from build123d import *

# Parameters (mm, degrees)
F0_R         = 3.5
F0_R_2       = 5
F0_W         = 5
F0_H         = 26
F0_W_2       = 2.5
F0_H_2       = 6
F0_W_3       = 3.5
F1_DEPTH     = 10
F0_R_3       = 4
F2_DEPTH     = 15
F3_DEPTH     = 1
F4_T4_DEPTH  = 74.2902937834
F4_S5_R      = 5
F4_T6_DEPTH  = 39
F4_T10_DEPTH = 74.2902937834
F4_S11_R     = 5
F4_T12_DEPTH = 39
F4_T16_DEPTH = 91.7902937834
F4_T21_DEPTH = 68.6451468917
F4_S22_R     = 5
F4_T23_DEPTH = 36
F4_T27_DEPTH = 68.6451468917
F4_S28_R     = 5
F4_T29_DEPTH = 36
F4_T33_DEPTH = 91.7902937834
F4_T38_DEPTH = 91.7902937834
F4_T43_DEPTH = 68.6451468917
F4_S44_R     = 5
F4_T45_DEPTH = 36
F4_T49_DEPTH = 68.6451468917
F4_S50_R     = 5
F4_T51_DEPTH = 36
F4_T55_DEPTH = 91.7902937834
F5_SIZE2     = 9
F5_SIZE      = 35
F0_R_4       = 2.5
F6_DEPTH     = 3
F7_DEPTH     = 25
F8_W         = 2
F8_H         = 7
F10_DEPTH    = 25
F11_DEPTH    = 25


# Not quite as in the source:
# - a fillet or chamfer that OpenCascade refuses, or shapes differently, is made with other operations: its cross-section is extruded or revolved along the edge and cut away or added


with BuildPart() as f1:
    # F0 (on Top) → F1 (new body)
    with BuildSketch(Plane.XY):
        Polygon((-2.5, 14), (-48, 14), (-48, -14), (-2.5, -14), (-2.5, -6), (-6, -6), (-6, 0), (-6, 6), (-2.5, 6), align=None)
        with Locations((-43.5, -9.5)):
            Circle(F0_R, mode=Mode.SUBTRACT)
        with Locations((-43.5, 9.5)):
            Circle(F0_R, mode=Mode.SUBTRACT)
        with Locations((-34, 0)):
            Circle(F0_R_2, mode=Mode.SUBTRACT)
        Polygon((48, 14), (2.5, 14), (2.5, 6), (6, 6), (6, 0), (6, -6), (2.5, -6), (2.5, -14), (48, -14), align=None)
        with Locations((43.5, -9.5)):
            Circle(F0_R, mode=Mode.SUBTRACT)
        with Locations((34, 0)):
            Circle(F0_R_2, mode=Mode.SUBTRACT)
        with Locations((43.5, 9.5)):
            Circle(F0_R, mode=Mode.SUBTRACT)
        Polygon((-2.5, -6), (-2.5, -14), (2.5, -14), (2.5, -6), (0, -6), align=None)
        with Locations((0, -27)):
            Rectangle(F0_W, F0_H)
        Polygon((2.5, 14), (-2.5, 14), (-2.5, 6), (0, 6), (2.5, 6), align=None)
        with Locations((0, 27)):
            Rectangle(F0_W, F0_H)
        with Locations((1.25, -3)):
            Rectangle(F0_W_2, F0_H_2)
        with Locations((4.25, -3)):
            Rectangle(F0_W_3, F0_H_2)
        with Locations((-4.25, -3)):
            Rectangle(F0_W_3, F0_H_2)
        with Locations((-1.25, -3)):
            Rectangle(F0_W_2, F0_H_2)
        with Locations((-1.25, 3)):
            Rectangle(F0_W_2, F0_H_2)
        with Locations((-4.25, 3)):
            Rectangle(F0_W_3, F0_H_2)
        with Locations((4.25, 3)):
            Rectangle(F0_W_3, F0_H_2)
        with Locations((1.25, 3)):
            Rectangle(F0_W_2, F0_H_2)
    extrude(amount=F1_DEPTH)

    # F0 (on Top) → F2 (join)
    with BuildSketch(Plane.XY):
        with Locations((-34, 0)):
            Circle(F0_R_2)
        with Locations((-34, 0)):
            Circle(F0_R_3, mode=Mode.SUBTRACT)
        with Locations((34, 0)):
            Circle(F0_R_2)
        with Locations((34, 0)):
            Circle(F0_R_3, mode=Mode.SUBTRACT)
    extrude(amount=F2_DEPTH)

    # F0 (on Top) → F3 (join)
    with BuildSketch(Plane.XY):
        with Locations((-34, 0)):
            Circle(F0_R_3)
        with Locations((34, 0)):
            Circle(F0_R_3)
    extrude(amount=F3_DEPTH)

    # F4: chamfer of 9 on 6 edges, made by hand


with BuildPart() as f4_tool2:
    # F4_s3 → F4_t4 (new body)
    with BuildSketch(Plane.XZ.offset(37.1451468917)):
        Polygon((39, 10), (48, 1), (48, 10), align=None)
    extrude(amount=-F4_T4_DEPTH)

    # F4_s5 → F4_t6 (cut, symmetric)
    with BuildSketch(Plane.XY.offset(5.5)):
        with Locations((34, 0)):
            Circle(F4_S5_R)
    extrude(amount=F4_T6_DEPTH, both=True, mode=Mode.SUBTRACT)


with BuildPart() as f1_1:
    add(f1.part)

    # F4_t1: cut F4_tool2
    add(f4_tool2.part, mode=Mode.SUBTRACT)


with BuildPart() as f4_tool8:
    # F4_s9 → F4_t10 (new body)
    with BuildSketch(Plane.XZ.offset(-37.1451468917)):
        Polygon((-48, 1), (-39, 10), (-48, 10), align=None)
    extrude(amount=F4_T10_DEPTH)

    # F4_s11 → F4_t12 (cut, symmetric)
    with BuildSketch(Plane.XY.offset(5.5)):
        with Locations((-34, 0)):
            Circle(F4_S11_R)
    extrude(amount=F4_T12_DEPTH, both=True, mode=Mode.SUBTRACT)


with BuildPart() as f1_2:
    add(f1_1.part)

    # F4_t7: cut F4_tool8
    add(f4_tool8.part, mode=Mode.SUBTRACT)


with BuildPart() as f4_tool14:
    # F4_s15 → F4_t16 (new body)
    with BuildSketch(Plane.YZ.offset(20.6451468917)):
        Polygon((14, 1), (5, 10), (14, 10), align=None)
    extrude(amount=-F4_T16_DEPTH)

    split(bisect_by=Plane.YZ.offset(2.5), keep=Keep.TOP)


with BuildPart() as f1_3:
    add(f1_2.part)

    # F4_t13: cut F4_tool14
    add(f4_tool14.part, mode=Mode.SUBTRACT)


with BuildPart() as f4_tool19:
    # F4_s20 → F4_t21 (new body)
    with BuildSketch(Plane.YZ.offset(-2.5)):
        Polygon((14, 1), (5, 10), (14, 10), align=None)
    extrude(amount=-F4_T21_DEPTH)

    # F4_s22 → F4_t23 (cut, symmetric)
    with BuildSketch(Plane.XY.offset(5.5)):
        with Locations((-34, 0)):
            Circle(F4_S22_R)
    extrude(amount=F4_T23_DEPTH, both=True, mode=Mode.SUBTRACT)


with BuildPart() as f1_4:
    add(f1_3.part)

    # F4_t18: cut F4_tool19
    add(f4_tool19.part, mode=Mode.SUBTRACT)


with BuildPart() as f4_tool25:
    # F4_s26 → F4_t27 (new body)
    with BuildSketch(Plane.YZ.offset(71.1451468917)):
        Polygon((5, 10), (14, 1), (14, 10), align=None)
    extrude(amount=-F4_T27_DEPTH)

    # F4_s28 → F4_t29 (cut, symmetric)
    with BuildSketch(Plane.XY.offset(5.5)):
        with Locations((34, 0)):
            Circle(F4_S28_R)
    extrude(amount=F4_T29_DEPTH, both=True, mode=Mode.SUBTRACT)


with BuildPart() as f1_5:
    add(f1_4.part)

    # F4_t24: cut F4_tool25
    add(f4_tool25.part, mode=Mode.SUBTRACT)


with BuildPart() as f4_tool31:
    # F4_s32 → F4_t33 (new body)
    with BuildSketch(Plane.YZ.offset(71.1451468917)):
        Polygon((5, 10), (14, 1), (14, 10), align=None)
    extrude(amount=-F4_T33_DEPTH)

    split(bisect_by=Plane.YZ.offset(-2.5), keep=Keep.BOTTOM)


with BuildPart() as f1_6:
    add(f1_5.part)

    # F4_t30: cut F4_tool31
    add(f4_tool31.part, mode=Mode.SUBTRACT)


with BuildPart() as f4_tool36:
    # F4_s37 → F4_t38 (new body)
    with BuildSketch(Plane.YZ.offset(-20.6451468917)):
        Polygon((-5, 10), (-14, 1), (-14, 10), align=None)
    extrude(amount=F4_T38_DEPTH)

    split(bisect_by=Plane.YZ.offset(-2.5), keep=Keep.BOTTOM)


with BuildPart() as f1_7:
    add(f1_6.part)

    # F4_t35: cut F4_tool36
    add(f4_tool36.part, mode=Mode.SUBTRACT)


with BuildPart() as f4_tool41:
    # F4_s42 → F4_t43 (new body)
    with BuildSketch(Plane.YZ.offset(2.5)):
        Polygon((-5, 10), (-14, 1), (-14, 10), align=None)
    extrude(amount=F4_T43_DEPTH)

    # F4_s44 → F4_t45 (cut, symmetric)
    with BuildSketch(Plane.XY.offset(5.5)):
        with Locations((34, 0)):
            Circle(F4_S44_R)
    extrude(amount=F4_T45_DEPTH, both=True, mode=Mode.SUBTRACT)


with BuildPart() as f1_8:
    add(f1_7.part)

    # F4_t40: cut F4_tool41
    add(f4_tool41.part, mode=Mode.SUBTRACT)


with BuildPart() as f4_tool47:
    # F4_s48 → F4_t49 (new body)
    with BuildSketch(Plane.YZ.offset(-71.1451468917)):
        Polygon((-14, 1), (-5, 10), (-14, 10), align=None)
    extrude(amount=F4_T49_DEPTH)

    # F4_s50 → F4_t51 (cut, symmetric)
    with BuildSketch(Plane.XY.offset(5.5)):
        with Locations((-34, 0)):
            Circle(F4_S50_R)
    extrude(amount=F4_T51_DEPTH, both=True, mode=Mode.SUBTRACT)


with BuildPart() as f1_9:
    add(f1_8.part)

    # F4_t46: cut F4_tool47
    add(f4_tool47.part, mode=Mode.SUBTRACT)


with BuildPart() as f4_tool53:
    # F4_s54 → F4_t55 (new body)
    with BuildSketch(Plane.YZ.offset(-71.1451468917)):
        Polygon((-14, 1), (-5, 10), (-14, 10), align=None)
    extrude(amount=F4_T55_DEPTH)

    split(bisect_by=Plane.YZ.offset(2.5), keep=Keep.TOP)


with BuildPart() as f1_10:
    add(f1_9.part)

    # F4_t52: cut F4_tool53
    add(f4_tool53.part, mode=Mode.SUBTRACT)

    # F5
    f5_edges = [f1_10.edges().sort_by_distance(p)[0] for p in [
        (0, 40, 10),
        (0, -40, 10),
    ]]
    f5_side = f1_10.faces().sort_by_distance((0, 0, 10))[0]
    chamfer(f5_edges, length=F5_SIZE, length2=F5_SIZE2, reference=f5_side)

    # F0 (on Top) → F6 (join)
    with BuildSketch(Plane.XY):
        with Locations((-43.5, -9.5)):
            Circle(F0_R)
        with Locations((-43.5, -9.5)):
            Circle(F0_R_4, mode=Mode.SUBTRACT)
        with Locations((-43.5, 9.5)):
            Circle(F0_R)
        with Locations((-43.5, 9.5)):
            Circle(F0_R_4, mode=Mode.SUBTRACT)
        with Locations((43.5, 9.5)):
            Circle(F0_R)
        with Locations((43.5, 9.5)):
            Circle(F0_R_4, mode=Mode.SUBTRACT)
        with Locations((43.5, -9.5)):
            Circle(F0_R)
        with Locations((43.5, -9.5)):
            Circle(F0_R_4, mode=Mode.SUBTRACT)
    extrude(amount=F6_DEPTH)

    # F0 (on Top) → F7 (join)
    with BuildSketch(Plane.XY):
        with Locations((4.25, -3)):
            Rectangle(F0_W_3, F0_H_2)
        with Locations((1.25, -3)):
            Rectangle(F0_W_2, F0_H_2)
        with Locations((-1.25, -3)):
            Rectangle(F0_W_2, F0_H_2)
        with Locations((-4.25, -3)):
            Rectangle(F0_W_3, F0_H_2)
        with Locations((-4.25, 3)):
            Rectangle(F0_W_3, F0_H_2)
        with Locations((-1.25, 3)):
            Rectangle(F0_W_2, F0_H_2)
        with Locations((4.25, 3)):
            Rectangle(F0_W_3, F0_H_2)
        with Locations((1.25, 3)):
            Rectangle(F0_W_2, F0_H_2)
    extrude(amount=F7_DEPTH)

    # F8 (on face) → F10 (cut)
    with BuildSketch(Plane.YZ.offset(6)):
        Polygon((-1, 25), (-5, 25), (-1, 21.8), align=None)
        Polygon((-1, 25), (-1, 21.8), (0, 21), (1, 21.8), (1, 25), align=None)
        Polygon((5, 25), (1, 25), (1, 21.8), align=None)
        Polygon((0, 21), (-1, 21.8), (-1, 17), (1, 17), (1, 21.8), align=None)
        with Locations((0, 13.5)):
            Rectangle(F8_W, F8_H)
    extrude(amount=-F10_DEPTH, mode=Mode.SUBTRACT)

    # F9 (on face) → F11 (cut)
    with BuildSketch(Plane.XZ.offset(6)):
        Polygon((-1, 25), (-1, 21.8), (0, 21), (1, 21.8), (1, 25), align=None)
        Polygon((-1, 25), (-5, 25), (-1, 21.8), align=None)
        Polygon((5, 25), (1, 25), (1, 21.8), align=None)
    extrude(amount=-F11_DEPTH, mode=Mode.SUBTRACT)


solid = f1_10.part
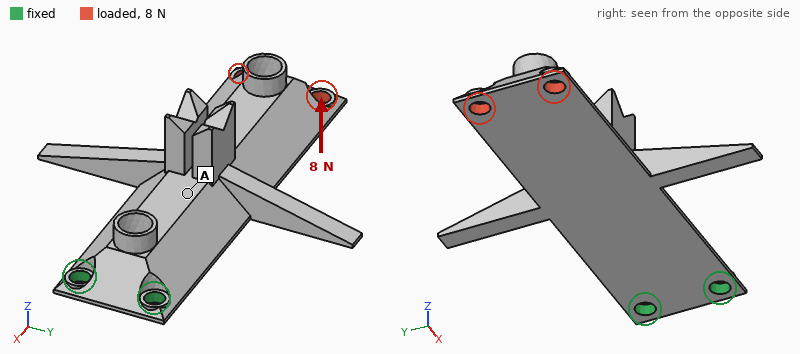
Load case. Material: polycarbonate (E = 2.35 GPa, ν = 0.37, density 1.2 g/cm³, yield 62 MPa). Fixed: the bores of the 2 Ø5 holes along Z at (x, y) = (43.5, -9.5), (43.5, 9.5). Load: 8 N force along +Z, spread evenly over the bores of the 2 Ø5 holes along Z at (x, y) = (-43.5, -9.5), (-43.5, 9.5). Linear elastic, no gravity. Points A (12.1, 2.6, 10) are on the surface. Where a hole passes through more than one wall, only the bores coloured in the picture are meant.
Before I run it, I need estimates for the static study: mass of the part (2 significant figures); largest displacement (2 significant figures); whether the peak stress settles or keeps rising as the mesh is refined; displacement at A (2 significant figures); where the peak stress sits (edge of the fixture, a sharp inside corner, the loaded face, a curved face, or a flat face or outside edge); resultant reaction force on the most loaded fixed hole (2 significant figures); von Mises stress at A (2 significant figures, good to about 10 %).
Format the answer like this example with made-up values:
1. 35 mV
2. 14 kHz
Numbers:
1. 24 g
2. 1.3 mm
3. keeps rising
4. 0.36 mm
5. edge of the fixture
6. 5.9 N
7. 1.7 MPa
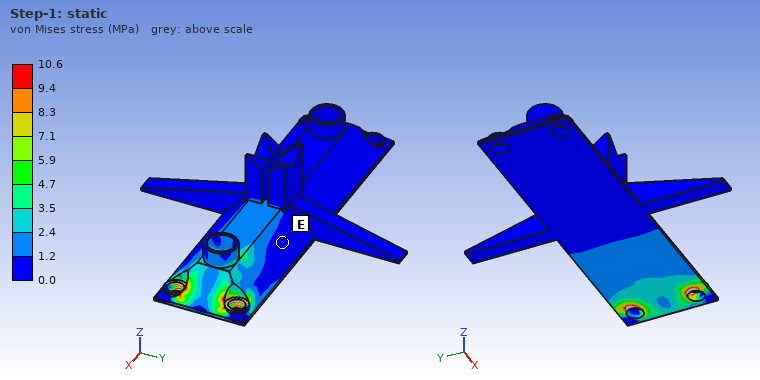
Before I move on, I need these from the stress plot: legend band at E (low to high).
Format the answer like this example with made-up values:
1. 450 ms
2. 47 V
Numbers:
1. 0.0 to 1.2 MPa
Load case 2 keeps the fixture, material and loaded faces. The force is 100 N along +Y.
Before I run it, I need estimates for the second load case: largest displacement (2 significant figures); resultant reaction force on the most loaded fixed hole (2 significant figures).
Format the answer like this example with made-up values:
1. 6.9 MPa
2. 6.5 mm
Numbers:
1. 1.5 mm
2. 430 N
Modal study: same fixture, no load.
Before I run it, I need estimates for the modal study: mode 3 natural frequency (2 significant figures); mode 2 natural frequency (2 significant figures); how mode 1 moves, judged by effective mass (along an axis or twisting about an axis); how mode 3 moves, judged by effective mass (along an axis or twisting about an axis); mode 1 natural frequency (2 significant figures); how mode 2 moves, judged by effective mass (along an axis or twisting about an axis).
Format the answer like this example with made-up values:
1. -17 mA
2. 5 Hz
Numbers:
1. 960 Hz
2. 580 Hz
3. along Z
4. twisting about X
5. 160 Hz
6. along Y
